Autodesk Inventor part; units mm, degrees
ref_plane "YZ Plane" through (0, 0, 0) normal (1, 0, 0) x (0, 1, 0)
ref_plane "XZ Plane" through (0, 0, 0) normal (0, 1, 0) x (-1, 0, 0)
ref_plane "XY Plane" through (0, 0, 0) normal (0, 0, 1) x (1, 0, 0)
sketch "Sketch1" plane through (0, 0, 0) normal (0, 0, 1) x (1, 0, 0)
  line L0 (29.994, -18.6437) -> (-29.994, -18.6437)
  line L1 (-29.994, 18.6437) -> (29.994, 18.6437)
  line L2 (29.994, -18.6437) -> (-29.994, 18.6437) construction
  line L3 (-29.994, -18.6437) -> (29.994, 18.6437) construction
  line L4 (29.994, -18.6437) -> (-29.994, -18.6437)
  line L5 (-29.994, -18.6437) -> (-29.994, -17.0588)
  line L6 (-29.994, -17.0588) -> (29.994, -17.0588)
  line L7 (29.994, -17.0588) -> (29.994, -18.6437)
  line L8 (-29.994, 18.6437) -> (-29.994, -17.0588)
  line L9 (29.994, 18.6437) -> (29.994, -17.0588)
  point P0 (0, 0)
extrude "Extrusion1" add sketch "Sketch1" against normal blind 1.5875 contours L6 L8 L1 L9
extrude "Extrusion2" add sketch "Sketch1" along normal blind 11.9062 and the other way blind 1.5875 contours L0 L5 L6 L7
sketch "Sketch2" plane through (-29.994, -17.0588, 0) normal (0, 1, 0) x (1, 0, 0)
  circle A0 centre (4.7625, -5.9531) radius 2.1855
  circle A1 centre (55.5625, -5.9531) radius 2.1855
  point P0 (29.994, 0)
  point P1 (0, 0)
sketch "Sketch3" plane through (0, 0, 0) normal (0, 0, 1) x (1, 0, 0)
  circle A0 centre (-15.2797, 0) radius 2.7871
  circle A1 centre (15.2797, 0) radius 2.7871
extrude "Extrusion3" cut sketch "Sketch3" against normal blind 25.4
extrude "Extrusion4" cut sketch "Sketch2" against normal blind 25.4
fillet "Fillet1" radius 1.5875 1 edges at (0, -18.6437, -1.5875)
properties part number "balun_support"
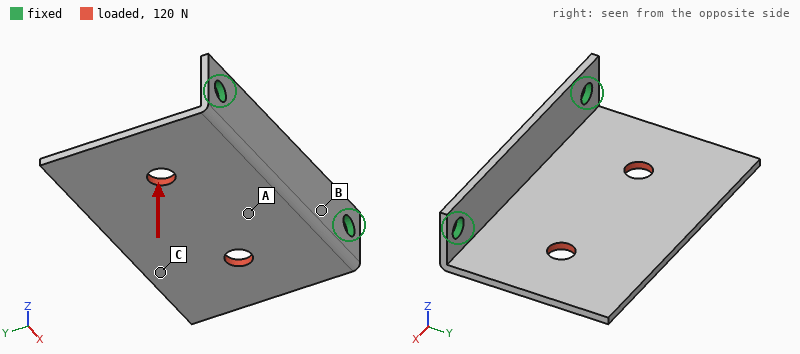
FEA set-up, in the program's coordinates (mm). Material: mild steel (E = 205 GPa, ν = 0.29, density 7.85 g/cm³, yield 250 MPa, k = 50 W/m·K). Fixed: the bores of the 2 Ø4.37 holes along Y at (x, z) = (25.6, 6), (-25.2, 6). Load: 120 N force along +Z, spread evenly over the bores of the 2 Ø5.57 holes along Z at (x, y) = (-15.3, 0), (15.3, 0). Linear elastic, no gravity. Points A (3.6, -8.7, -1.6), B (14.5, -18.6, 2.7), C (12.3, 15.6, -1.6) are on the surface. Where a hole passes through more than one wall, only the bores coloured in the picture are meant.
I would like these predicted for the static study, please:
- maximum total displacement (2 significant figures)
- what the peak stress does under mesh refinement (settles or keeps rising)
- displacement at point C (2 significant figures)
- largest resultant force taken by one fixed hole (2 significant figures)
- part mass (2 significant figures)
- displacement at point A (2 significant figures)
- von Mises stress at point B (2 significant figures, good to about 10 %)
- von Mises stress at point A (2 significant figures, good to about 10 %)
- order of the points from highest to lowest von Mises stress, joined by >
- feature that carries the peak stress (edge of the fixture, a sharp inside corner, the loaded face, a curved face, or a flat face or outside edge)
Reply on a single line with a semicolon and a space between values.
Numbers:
0.32 mm; keeps rising; 0.29 mm; 62 N; 36 g; 0.068 mm; 70 MPa; 32 MPa; B > A > C; edge of the fixture
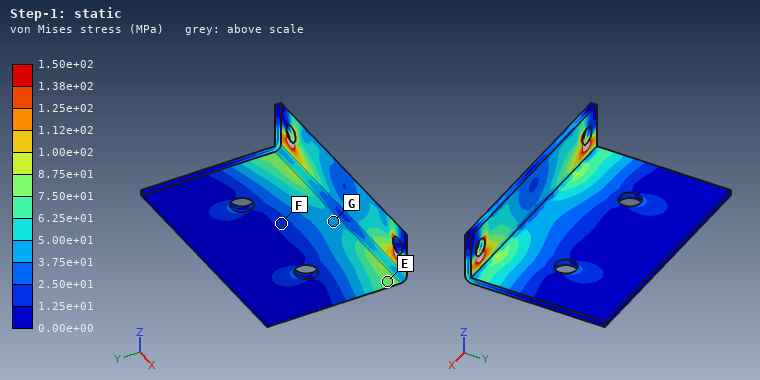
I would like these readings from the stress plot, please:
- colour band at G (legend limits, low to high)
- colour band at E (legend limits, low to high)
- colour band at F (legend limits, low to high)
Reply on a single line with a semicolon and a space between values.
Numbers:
3.75e+01 to 5.00e+01 MPa; 7.50e+01 to 8.75e+01 MPa; 1.25e+01 to 2.50e+01 MPa
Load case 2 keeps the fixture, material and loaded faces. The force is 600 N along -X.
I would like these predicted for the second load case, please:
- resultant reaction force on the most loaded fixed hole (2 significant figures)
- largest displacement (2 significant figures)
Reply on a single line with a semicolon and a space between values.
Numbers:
370 N; 46 µm
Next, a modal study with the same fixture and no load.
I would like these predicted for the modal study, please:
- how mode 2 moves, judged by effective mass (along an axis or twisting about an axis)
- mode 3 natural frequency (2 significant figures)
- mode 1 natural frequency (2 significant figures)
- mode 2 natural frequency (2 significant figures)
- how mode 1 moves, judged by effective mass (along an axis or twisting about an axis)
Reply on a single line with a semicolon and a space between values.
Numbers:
twisting about Y; 3500 Hz; 700 Hz; 1500 Hz; along Z
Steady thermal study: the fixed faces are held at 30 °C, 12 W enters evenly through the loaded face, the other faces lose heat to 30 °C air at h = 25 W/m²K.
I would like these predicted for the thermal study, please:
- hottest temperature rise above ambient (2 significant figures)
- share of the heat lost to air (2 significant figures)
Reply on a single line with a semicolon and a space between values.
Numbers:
62 K; 44 %
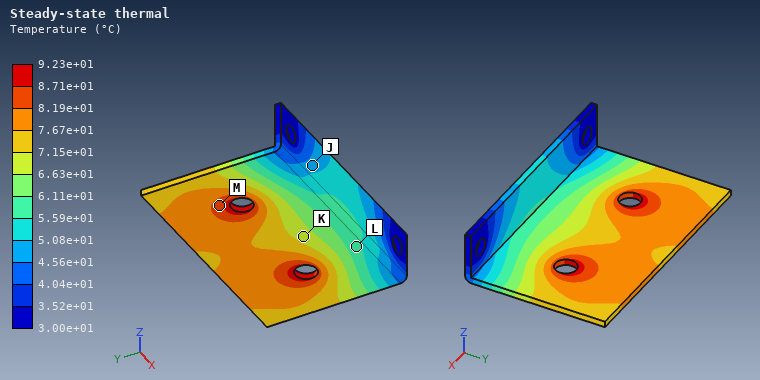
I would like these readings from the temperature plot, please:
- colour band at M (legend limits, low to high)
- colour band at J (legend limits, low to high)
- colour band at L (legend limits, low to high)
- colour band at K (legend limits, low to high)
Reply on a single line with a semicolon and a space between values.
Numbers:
8.19e+01 to 8.71e+01 °C; 4.56e+01 to 5.08e+01 °C; 5.59e+01 to 6.11e+01 °C; 6.63e+01 to 7.15e+01 °C
